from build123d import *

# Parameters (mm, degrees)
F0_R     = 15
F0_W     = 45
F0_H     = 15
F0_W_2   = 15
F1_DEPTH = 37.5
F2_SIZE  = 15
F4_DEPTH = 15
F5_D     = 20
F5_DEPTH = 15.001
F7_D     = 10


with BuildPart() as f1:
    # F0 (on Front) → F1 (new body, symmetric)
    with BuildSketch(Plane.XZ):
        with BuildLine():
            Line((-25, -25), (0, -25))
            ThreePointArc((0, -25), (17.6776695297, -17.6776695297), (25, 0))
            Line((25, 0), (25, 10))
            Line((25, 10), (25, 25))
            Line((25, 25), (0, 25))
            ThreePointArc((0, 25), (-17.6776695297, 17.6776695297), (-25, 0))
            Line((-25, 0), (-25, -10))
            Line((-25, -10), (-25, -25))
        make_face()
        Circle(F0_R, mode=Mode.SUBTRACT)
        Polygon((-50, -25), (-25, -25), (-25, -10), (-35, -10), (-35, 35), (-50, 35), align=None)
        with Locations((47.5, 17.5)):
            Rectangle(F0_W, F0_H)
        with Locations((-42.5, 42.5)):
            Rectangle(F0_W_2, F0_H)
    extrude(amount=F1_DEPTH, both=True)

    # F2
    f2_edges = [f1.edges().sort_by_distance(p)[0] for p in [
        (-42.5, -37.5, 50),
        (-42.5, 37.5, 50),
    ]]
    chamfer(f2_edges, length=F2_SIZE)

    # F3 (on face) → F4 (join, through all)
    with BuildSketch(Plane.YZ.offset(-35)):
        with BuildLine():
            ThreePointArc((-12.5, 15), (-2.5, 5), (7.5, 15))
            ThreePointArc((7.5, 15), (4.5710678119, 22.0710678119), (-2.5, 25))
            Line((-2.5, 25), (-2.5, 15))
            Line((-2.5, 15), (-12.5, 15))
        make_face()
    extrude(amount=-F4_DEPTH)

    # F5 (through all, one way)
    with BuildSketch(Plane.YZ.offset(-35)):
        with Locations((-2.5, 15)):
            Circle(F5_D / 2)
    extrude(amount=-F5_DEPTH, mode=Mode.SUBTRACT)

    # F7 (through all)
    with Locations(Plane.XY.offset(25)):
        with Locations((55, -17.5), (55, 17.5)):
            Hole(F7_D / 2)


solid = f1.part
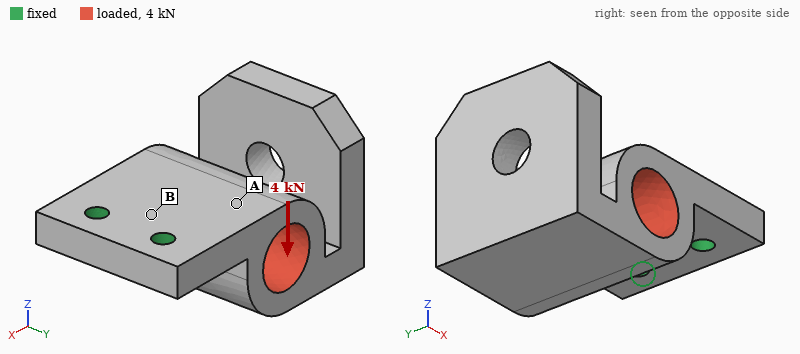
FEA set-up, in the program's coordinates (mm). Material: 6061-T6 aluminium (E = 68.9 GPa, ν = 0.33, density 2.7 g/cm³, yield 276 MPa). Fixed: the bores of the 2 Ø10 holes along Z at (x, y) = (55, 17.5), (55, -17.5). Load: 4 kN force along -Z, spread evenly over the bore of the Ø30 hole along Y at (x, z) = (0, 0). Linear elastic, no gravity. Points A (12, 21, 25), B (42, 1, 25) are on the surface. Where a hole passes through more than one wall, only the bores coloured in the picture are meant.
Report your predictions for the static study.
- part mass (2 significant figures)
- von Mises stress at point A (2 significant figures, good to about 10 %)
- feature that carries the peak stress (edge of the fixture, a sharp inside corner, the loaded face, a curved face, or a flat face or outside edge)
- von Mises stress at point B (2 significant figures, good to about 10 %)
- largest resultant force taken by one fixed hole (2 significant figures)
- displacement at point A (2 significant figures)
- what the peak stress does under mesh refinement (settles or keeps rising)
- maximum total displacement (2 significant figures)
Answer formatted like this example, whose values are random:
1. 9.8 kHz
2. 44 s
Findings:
1. 680 g
2. 15 MPa
3. edge of the fixture
4. 47 MPa
5. 2.0 kN
6. 0.11 mm
7. keeps rising
8. 0.38 mm
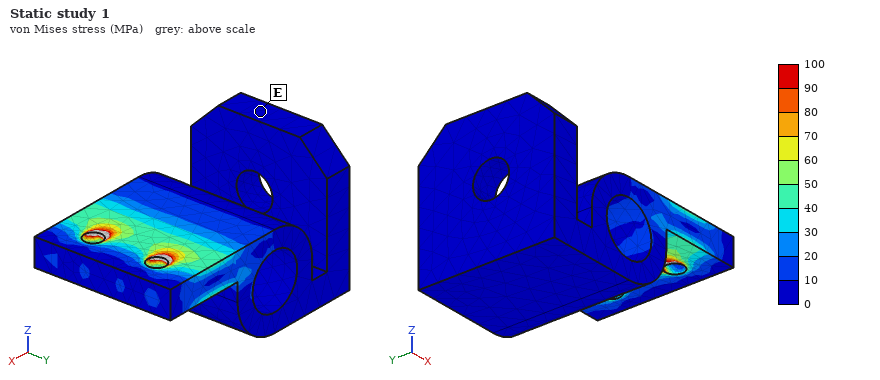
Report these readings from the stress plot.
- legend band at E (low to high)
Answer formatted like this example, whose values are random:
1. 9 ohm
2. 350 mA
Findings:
1. 0 to 10 MPa
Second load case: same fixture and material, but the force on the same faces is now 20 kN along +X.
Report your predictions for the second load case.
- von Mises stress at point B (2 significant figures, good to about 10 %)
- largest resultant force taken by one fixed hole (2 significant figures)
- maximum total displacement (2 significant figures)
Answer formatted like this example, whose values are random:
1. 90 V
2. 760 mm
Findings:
1. 87 MPa
2. 10 kN
3. 0.90 mm
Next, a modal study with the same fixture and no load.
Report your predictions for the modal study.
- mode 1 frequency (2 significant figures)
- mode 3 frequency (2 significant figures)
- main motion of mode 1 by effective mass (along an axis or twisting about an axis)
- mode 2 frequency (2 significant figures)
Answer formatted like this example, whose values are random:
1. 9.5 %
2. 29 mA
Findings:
1. 640 Hz
2. 1800 Hz
3. along Z
4. 1800 Hz
